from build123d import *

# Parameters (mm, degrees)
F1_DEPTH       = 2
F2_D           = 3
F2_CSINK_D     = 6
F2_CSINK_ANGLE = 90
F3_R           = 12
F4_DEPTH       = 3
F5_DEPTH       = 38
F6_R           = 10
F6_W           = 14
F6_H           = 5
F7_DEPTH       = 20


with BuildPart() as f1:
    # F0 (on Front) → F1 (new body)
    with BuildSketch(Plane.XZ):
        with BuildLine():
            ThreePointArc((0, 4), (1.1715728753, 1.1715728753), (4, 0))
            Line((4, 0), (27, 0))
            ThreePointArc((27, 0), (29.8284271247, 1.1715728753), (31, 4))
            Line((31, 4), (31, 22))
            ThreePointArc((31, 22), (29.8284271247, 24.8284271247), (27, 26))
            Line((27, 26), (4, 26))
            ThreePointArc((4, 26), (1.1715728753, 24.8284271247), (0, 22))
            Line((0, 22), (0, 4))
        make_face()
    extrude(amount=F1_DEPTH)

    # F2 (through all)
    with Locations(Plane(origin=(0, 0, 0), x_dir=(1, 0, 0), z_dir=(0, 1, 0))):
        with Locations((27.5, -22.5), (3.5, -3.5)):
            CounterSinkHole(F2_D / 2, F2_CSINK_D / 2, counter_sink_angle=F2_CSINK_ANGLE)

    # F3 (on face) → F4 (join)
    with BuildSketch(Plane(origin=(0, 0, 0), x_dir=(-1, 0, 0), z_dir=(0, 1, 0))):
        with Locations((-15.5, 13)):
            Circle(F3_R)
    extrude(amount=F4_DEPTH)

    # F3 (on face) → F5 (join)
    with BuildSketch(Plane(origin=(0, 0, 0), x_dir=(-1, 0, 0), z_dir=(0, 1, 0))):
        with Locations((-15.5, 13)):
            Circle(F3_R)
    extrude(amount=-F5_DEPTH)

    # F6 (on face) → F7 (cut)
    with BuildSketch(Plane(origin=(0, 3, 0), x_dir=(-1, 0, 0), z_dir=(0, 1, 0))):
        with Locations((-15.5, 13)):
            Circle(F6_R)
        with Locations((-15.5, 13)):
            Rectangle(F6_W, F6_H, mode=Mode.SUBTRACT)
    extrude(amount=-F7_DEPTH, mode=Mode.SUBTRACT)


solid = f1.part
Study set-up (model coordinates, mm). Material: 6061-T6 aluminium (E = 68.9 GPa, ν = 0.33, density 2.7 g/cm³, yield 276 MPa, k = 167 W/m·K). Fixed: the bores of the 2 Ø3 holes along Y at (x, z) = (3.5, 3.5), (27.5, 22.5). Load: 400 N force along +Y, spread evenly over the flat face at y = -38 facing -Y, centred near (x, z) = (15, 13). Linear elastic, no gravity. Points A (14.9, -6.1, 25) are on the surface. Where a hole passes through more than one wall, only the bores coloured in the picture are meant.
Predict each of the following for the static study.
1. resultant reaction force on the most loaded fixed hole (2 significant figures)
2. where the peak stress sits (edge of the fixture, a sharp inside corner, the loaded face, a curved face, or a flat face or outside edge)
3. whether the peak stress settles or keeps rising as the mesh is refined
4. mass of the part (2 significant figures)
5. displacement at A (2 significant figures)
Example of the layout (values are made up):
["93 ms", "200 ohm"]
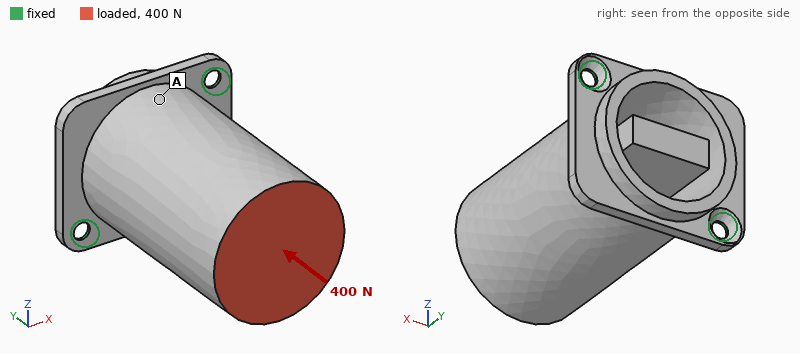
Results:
["200 N", "edge of the fixture", "keeps rising", "39 g", "10 µm"]
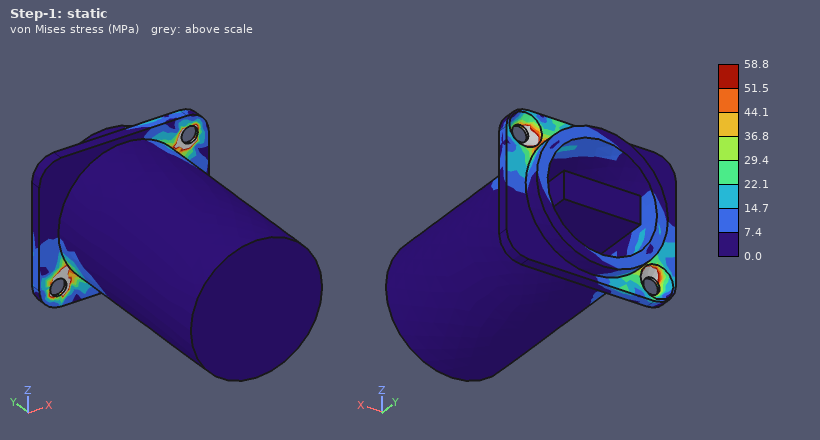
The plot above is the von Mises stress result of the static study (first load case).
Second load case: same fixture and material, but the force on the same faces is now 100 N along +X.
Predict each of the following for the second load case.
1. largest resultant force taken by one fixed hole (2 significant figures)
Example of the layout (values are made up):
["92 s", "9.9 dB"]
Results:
["120 N"]
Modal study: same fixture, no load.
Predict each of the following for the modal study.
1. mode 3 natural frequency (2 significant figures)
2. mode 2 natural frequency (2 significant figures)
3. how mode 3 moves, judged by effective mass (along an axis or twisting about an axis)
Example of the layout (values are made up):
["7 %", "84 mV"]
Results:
["5000 Hz", "2800 Hz", "along Y"]
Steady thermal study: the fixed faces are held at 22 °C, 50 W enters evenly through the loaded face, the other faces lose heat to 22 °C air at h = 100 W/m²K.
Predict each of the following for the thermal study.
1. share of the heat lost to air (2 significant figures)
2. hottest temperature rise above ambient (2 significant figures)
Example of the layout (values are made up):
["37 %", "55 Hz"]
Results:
["50 %", "61 K"]
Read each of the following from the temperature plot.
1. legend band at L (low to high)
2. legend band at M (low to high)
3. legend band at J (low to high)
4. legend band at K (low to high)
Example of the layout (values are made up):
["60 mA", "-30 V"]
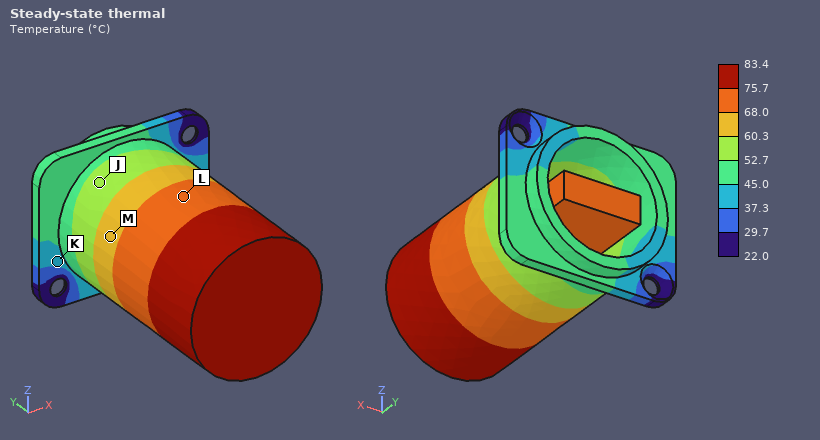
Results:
["68.0 to 75.7 °C", "60.3 to 68.0 °C", "52.7 to 60.3 °C", "37.3 to 45.0 °C"]
